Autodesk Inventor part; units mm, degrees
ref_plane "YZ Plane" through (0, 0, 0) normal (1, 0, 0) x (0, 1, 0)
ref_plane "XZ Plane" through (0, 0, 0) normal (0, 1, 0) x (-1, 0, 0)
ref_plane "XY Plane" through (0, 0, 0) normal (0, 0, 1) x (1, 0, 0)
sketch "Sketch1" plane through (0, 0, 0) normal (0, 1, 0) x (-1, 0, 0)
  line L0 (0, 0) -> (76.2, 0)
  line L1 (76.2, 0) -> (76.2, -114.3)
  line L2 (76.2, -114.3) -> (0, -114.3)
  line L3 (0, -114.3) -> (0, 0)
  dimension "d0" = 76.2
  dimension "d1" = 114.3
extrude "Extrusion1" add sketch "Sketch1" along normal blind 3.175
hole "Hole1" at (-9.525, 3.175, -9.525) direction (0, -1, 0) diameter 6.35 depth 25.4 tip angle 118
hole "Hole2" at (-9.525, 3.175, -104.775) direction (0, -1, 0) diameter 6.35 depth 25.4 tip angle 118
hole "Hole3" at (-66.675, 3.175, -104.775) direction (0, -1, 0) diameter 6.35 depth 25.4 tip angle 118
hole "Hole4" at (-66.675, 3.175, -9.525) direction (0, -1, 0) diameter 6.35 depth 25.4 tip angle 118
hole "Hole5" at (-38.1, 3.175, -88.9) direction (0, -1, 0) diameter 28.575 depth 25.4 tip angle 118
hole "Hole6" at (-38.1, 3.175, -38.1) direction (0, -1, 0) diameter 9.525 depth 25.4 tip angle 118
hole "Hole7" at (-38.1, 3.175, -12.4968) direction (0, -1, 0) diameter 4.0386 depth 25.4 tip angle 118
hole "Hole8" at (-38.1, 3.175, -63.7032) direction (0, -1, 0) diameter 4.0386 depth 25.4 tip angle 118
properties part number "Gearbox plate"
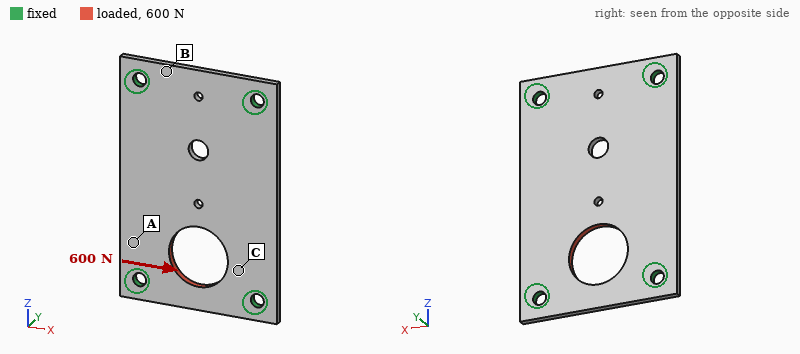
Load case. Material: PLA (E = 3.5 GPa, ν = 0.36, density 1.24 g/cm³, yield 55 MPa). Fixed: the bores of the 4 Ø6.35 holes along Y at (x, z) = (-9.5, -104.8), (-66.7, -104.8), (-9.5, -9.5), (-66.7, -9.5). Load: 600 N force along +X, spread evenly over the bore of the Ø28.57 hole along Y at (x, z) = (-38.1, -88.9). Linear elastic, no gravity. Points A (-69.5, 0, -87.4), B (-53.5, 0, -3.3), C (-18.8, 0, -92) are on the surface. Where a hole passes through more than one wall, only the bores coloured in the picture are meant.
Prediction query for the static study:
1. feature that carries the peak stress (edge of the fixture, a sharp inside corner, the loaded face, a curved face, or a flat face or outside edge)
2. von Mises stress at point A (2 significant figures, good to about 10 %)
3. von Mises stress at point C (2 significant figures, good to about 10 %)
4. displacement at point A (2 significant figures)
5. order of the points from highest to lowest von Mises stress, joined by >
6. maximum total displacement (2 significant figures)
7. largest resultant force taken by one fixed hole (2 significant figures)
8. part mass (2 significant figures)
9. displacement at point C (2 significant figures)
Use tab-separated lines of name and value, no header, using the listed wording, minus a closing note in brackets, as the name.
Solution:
feature that carries the peak stress	edge of the fixture
von Mises stress at point A	1.9 MPa
von Mises stress at point C	3.4 MPa
displacement at point A	36 µm
order of the points from highest to lowest von Mises stress, joined by >	C > A > B
maximum total displacement	57 µm
largest resultant force taken by one fixed hole	230 N
part mass	31 g
displacement at point C	31 µm
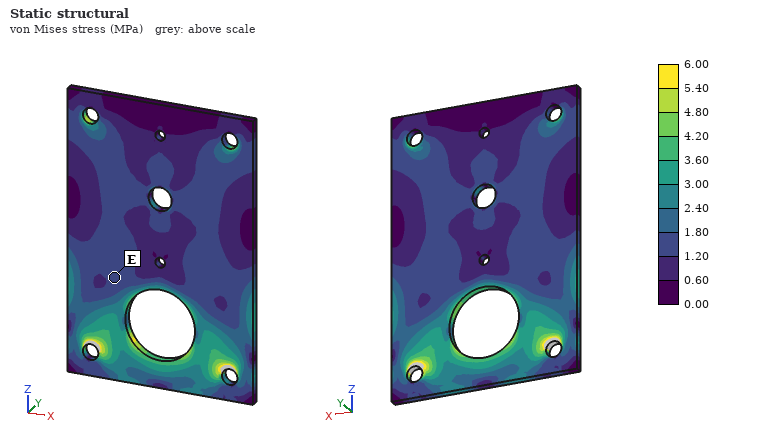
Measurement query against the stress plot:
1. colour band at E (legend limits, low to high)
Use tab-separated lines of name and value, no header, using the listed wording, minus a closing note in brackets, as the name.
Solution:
colour band at E	1.20 to 1.80 MPa
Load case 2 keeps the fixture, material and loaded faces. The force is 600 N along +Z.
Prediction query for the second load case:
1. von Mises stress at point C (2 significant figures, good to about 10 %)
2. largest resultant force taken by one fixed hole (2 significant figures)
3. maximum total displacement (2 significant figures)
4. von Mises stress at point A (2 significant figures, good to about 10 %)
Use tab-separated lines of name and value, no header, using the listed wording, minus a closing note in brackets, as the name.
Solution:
von Mises stress at point C	3.7 MPa
largest resultant force taken by one fixed hole	210 N
maximum total displacement	66 µm
von Mises stress at point A	1.9 MPa
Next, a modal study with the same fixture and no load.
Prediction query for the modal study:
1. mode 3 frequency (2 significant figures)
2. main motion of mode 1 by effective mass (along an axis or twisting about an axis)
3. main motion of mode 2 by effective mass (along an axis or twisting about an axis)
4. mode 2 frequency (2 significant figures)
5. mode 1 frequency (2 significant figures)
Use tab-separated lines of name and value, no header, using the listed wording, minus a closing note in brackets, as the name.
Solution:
mode 3 frequency	1300 Hz
main motion of mode 1 by effective mass	along Y
main motion of mode 2 by effective mass	twisting about Z
mode 2 frequency	800 Hz
mode 1 frequency	580 Hz
